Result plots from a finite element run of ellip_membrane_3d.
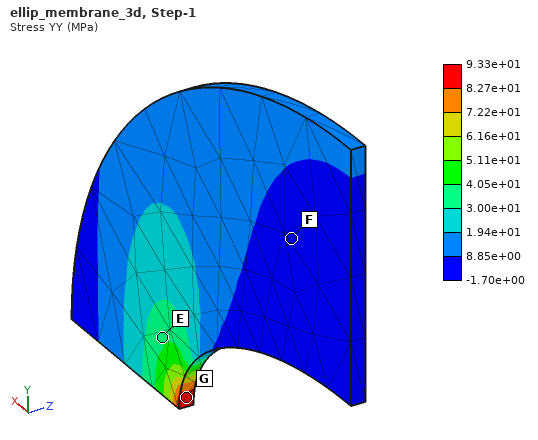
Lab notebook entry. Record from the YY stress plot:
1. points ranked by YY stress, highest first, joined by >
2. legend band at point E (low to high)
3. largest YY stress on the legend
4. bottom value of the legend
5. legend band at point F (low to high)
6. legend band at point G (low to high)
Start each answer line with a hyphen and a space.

- G > E > F
- 3.00e+01 to 4.05e+01 MPa
- 9.33e+01 MPa
- -1.70e+00 MPa
- -1.70e+00 to 8.85e+00 MPa
- 8.27e+01 to 9.33e+01 MPa
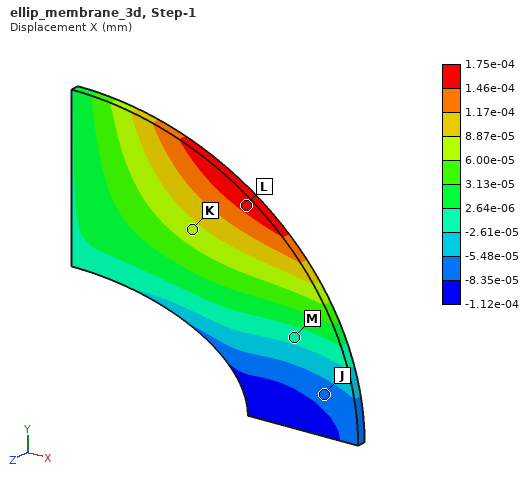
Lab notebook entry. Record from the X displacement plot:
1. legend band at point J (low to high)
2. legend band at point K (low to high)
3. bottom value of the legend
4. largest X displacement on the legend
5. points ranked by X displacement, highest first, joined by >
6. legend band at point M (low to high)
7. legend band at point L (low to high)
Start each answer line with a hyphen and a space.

- -8.35e-05 to -5.48e-05 mm
- 6.00e-05 to 8.87e-05 mm
- -1.12e-04 mm
- 1.75e-04 mm
- L > K > M > J
- -2.61e-05 to 2.64e-06 mm
- 1.46e-04 to 1.75e-04 mm
